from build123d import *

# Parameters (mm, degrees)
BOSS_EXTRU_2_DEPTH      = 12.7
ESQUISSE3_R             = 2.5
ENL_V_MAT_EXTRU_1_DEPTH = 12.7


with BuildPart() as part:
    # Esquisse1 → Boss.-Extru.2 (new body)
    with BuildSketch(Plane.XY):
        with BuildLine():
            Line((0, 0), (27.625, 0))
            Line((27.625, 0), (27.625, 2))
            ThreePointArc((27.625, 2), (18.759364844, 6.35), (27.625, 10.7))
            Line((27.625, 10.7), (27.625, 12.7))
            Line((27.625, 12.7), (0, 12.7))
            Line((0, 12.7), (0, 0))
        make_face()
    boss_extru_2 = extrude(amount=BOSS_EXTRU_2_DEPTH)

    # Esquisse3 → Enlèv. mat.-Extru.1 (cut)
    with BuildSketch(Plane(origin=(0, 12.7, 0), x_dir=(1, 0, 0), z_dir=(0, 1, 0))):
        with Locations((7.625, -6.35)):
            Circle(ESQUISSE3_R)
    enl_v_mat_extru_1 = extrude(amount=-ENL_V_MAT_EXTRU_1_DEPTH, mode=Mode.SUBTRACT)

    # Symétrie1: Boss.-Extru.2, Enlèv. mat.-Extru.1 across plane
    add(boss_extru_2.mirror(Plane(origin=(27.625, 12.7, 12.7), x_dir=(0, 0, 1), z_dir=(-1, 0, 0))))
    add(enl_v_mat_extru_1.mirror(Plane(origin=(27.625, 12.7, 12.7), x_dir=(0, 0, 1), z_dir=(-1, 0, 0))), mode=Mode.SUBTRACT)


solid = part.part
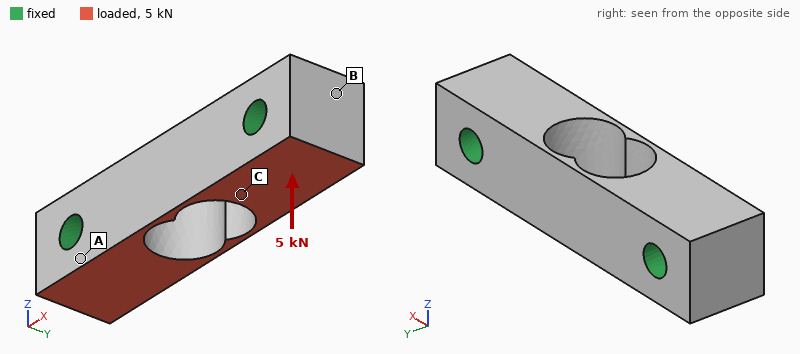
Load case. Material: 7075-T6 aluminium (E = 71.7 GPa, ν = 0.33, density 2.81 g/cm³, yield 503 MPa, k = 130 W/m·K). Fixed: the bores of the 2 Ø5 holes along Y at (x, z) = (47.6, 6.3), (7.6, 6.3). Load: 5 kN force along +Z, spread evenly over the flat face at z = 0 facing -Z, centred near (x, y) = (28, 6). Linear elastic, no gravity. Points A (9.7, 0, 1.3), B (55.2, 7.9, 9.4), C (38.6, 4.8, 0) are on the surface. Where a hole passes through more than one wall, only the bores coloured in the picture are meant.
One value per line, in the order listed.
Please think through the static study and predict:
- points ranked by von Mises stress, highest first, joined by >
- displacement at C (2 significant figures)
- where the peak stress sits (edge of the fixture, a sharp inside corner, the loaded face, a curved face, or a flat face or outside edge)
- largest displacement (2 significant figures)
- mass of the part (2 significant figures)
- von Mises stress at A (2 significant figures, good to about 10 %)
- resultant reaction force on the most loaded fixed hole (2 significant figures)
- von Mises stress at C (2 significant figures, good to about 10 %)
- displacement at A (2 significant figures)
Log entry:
A > C > B
6.0 µm
edge of the fixture
9.6 µm
18 g
19 MPa
2.5 kN
11 MPa
1.7 µm
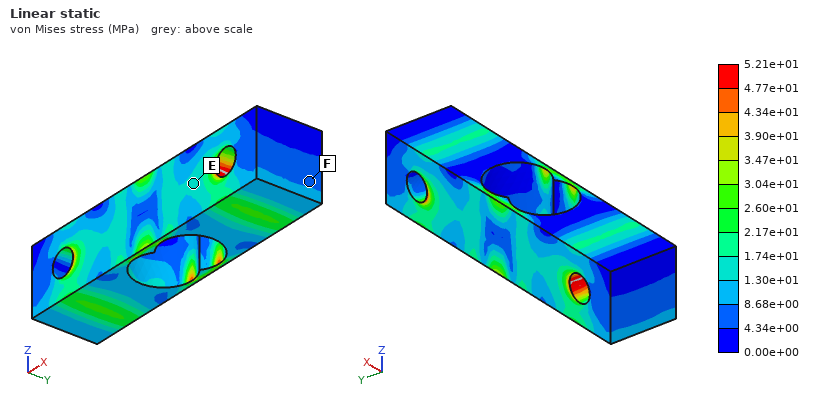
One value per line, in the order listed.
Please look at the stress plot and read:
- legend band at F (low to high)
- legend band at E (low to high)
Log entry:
4.34e+00 to 8.68e+00 MPa
1.30e+01 to 1.74e+01 MPa
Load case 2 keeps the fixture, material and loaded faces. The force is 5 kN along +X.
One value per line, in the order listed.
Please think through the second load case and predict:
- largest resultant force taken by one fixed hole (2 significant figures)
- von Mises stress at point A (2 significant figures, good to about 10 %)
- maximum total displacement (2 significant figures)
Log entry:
2.5 kN
21 MPa
5.6 µm
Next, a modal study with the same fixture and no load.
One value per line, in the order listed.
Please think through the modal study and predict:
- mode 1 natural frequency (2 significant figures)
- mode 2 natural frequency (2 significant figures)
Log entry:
30 kHz
32 kHz
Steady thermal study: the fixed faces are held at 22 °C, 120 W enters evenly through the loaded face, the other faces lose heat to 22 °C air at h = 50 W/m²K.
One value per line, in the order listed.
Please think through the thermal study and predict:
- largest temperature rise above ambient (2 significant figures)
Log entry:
23 K
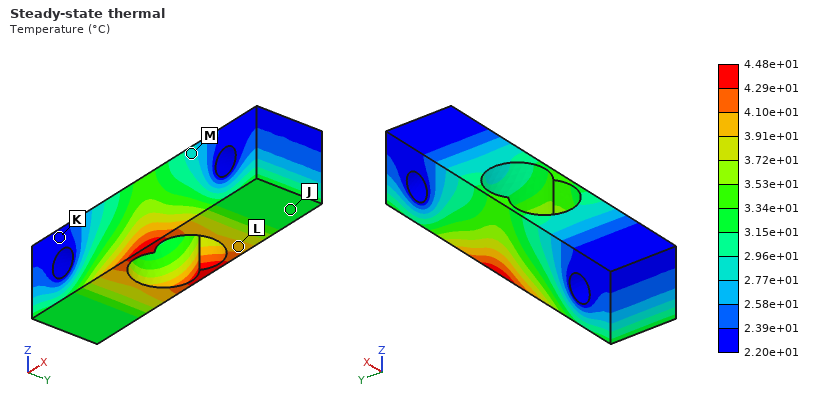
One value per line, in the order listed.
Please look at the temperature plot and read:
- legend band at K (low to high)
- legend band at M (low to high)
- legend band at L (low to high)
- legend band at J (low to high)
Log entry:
2.20e+01 to 2.39e+01 °C
2.77e+01 to 2.96e+01 °C
3.91e+01 to 4.10e+01 °C
3.15e+01 to 3.34e+01 °C
